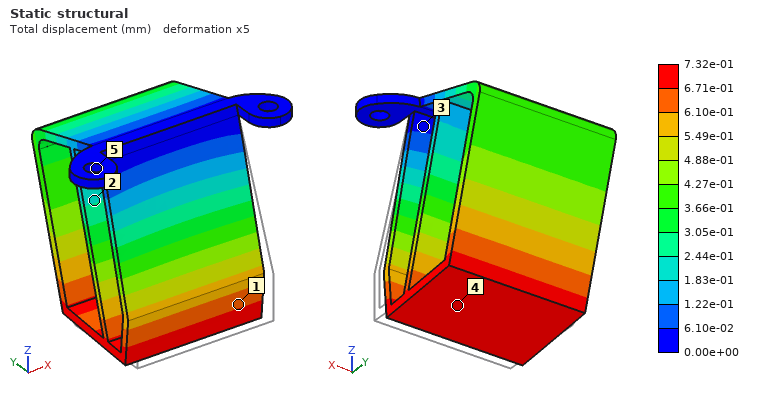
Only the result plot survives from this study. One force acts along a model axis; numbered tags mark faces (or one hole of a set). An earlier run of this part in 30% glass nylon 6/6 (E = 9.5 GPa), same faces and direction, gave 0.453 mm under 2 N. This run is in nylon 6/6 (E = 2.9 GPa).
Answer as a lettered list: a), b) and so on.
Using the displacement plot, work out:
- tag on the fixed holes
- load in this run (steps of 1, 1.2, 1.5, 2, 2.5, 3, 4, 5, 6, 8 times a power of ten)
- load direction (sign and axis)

a) 5
b) 1 N
c) +Y
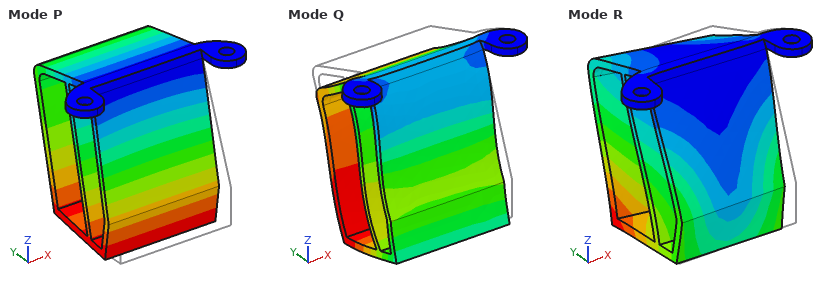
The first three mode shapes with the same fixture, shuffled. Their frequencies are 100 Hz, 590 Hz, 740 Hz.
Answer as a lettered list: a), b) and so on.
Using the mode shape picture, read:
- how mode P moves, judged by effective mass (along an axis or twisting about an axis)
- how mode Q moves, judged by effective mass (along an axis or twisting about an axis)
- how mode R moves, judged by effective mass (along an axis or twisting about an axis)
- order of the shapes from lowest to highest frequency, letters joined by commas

a) along Y
b) along Z
c) along X
d) P, R, Q
